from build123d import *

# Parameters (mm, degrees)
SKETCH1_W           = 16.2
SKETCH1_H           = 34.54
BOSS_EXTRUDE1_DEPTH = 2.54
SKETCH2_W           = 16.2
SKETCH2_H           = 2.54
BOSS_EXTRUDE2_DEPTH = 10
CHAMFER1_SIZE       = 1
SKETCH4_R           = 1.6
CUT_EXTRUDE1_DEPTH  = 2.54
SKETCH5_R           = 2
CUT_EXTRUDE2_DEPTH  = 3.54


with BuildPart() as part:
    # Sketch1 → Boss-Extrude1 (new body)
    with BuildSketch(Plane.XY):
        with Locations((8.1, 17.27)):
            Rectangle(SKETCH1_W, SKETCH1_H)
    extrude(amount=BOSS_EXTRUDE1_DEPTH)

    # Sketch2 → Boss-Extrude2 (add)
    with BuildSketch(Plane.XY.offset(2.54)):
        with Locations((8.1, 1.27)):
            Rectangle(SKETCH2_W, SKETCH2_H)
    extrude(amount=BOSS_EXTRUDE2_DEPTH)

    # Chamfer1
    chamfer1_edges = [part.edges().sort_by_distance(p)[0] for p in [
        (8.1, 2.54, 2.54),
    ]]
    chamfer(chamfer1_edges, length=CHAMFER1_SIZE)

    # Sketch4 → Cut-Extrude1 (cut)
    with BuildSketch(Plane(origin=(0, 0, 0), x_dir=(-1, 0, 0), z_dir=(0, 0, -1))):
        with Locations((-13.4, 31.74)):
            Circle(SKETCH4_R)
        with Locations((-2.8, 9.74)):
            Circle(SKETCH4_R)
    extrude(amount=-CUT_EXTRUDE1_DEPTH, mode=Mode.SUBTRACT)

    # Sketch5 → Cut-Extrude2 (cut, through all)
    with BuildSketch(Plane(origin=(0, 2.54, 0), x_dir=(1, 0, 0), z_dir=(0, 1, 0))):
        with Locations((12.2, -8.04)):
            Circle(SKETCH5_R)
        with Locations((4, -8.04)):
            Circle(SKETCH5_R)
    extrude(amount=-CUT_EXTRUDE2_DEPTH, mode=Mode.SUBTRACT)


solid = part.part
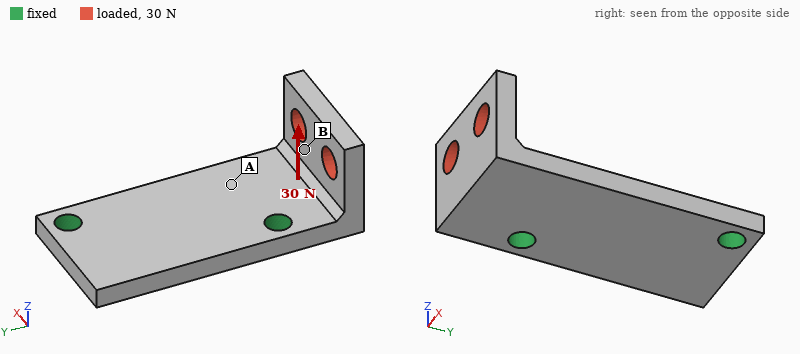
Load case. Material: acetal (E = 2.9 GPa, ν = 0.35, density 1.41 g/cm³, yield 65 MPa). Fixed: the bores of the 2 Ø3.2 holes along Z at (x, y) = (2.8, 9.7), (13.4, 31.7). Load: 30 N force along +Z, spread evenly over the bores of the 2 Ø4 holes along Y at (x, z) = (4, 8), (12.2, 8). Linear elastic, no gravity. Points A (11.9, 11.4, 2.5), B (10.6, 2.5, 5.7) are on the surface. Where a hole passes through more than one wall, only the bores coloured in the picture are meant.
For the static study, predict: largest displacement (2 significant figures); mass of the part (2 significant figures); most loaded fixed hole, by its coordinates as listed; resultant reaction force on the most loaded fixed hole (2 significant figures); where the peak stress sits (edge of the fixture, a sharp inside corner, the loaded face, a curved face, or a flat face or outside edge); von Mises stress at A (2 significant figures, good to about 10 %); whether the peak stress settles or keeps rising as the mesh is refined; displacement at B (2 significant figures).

0.37 mm
2.4 g
(2.8, 9.7)
33 N
edge of the fixture
5.9 MPa
keeps rising
0.19 mm
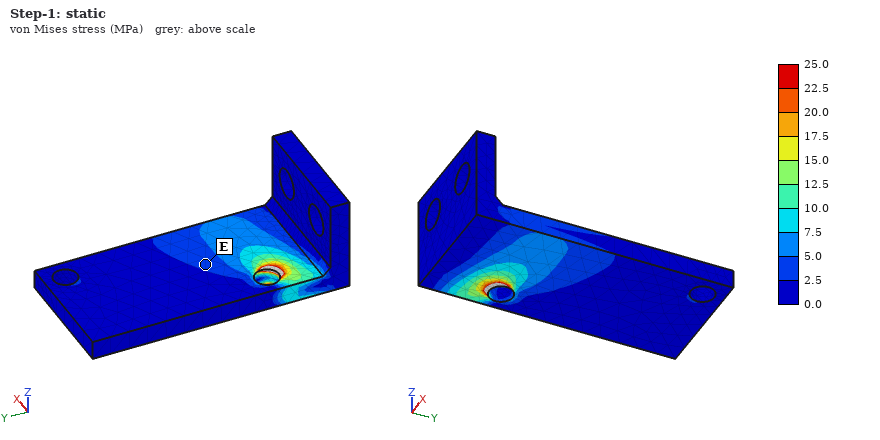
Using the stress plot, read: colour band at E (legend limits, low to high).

2.5 to 5.0 MPa
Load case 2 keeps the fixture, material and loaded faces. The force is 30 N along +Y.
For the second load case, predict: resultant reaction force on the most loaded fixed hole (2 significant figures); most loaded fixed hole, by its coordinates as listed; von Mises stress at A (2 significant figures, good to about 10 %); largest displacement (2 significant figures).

22 N
(2.8, 9.7)
5.7 MPa
0.41 mm
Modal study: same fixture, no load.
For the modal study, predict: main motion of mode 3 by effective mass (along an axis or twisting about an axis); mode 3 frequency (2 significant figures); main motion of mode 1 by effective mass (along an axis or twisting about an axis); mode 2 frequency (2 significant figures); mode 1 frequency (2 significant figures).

along Z
4100 Hz
along Z
2600 Hz
1800 Hz
